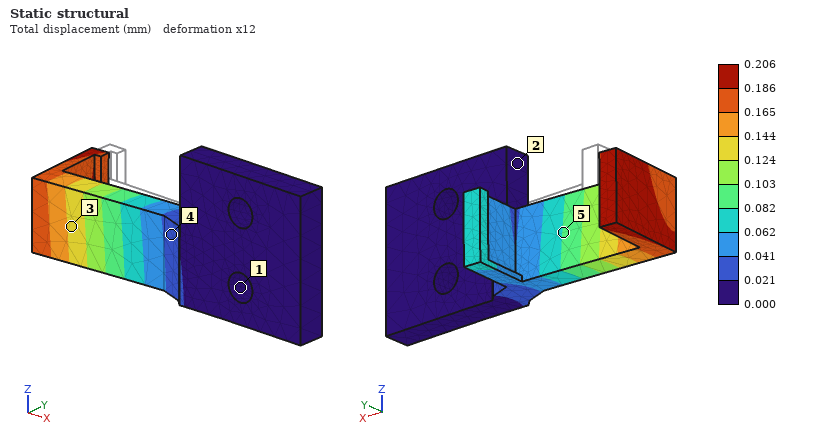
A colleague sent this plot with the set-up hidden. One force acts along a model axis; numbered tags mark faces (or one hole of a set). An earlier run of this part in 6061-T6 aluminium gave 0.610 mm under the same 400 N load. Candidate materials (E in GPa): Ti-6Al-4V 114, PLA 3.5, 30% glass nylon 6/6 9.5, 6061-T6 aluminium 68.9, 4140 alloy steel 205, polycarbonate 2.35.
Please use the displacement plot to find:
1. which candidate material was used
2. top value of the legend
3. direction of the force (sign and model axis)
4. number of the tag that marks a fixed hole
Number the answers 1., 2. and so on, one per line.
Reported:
1. 4140 alloy steel
2. 0.206 mm
3. -Y
4. 1
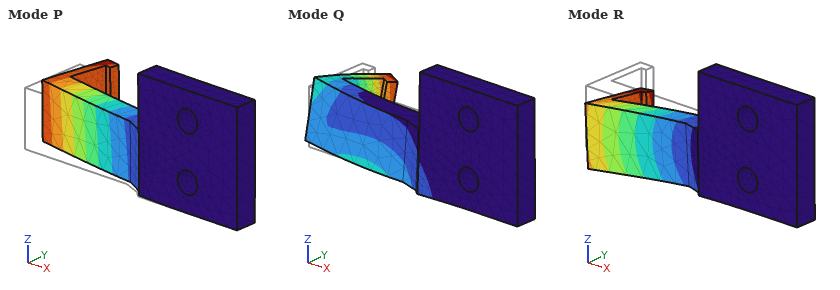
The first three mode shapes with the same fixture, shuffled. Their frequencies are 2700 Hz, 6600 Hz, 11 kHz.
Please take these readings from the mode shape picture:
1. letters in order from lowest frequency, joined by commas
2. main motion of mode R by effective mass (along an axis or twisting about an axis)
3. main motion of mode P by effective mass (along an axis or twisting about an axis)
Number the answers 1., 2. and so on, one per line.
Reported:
1. P, R, Q
2. along Z
3. along Y
